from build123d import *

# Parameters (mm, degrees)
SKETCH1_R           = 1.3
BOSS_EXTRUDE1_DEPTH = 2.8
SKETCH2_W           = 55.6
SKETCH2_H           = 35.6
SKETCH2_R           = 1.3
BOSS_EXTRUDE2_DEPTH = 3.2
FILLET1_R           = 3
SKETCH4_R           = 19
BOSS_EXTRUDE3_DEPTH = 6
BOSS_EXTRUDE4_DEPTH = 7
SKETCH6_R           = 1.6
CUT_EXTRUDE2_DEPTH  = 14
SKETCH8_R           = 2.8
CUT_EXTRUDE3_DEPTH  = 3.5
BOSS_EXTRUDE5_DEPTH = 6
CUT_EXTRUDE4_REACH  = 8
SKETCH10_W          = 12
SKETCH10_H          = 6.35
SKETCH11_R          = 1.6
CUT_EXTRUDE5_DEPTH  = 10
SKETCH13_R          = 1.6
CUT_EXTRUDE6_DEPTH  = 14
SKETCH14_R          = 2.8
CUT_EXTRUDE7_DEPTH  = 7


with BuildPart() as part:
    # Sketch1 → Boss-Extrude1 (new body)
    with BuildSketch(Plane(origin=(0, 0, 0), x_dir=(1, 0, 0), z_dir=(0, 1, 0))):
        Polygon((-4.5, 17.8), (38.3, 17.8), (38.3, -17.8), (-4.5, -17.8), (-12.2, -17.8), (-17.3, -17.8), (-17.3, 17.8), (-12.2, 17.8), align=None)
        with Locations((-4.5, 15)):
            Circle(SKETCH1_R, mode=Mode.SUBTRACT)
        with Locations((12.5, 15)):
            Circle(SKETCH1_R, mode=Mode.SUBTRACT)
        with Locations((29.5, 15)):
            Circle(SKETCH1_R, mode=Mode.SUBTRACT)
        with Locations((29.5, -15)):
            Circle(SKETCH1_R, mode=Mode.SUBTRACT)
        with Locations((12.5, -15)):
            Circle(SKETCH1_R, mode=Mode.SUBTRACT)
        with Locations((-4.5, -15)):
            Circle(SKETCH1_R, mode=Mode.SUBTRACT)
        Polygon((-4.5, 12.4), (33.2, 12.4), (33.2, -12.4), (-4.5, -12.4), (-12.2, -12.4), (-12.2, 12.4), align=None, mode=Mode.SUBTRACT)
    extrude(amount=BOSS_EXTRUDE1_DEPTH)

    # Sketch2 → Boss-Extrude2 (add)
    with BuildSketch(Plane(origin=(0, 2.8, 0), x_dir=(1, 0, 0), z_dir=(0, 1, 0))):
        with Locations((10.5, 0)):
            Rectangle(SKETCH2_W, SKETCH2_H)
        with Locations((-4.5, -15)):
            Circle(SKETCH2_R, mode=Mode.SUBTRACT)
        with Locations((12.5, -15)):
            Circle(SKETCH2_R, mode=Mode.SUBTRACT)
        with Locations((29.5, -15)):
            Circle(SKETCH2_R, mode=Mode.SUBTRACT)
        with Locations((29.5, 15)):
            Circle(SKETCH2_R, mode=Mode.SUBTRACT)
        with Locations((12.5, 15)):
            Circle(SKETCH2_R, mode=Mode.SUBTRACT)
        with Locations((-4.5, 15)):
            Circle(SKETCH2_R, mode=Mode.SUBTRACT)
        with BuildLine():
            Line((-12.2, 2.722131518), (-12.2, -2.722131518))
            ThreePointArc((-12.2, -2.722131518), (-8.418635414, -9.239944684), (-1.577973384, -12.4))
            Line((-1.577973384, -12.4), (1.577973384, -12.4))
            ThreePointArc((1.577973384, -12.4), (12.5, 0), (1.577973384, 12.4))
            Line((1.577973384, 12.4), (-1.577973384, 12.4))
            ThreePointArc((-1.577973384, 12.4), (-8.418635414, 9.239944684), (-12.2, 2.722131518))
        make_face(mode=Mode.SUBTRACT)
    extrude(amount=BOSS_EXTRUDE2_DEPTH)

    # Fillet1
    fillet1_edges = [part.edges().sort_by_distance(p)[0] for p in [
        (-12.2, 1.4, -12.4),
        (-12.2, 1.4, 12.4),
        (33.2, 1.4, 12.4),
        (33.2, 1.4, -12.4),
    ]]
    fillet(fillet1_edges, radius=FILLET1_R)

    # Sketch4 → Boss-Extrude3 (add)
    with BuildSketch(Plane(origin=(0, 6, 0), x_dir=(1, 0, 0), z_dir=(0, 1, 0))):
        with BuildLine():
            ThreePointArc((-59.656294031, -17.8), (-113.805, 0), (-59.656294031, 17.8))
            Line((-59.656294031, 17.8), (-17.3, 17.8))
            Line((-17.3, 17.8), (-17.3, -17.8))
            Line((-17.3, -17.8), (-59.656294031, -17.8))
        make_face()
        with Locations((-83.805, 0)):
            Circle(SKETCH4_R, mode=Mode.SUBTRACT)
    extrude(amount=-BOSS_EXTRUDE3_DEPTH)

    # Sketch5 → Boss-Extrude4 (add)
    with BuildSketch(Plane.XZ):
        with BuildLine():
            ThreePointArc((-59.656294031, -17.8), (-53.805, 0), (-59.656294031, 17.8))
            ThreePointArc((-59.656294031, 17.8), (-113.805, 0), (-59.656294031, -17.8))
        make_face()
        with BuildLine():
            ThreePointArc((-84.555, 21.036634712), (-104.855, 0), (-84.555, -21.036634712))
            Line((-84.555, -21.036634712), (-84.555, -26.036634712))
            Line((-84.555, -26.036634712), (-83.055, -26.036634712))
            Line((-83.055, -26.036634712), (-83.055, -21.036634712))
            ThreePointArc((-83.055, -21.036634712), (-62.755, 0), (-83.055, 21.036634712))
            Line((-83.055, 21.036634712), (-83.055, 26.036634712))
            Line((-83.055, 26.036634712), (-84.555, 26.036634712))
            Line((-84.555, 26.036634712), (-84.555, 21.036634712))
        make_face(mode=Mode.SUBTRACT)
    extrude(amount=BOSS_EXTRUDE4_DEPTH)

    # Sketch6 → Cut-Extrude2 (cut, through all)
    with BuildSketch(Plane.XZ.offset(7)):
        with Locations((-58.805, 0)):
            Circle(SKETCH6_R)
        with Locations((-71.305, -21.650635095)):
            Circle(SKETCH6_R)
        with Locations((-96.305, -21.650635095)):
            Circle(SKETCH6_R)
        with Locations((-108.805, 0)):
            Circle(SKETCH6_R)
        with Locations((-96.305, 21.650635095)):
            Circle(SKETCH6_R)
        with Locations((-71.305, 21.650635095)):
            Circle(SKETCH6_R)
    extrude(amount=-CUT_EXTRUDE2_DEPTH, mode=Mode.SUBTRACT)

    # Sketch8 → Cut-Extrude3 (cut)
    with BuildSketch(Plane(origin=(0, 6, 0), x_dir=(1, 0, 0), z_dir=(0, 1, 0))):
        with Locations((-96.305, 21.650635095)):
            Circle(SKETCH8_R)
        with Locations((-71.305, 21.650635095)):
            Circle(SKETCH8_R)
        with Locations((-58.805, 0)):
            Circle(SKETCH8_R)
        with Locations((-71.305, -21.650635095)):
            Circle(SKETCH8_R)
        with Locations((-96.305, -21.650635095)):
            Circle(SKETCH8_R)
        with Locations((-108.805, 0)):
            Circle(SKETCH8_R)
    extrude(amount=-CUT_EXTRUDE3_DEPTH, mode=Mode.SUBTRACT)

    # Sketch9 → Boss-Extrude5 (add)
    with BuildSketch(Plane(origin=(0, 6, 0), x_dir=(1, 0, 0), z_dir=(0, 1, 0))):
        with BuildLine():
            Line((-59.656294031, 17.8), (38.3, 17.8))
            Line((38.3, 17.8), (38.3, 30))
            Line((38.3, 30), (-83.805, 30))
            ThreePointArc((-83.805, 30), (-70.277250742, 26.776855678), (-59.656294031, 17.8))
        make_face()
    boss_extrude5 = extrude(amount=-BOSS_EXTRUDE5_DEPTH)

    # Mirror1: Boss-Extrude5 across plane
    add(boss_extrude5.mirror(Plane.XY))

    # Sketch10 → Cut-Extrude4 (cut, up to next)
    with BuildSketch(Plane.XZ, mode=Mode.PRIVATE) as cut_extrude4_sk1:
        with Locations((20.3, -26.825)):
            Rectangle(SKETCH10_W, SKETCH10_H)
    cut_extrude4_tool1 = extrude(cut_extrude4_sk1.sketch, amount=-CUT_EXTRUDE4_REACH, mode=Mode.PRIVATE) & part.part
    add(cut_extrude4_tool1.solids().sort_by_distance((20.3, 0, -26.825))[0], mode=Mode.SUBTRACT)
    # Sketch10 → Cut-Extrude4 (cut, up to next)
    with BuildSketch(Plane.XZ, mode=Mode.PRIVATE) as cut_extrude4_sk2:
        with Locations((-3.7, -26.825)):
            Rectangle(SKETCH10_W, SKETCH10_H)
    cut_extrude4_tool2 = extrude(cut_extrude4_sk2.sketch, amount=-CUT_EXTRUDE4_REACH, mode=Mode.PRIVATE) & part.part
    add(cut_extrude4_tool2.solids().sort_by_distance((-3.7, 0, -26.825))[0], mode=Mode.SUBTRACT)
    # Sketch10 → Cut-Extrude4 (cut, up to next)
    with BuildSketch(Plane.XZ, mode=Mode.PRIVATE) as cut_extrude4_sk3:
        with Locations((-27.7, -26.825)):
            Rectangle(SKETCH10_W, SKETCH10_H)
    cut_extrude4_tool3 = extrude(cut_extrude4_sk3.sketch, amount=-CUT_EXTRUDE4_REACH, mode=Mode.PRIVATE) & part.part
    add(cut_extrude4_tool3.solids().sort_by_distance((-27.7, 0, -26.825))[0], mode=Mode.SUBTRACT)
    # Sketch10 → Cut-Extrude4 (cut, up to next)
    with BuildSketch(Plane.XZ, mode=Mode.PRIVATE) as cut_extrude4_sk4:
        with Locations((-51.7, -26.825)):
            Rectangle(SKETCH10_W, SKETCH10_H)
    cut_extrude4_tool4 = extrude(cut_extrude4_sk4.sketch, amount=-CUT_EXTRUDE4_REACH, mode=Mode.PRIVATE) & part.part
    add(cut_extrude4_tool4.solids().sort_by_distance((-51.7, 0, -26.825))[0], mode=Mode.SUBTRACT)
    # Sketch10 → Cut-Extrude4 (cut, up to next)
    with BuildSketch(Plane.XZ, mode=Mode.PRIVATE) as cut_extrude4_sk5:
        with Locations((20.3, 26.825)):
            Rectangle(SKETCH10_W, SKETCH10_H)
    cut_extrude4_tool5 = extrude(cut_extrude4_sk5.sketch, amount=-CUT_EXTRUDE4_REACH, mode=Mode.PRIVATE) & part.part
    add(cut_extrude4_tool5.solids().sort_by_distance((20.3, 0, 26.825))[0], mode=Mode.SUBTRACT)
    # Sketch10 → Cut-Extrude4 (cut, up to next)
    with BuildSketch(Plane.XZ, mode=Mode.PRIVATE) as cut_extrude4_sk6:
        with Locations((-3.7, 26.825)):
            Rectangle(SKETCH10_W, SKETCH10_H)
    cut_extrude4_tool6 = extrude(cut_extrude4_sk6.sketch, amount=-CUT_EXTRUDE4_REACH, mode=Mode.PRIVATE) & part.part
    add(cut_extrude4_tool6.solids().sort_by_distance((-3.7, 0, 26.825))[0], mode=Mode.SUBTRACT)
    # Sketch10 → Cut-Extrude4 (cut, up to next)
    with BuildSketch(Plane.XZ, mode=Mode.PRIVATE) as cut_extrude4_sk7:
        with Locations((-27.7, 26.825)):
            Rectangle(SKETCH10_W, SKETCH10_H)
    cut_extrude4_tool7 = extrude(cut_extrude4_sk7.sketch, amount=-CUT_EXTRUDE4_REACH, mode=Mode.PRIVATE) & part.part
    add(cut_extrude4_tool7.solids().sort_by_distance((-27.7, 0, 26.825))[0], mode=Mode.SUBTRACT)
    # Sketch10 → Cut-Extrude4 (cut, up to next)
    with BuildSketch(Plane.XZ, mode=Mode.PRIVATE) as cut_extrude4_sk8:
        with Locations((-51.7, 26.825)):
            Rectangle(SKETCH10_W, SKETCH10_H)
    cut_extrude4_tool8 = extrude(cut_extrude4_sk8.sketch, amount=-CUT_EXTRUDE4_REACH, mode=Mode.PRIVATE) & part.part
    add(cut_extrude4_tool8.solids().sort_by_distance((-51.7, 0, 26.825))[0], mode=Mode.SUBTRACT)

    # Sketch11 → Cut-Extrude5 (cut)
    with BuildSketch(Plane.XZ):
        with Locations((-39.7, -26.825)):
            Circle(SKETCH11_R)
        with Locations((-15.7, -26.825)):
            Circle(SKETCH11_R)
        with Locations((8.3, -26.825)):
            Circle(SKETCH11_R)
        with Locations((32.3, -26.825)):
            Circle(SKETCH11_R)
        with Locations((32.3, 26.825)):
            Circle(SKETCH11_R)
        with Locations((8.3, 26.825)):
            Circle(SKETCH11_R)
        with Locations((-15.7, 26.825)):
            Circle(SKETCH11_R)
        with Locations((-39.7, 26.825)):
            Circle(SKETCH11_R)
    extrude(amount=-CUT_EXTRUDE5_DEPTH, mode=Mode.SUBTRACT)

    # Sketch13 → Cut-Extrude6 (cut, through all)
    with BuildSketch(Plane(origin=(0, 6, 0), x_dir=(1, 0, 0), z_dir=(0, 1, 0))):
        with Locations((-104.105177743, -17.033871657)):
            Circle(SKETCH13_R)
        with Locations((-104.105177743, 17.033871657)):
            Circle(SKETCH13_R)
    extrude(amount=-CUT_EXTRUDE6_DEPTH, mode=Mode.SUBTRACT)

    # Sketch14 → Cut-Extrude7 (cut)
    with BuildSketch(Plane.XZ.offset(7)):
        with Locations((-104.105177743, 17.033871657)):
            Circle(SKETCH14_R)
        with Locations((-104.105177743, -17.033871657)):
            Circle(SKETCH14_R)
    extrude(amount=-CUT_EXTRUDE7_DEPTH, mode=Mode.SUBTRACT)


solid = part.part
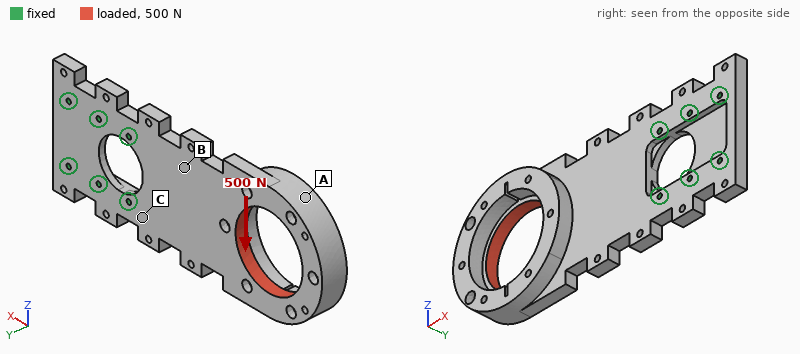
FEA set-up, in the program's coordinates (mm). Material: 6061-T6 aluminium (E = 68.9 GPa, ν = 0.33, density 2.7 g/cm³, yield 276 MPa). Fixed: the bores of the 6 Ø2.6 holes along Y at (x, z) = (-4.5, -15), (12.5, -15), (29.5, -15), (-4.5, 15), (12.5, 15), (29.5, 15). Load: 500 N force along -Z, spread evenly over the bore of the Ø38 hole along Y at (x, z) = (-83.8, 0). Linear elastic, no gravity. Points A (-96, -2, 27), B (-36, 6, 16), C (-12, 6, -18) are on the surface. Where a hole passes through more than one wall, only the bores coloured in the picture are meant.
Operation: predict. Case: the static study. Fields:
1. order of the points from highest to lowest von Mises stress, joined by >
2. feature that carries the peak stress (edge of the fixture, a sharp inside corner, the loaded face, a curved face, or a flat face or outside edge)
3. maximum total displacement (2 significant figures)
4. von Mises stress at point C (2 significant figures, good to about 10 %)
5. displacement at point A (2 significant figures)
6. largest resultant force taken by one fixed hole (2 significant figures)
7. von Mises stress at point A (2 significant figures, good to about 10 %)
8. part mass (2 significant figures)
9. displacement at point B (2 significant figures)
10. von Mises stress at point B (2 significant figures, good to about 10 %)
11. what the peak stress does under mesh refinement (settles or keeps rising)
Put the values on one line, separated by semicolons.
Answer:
C > B > A; edge of the fixture; 64 µm; 12 MPa; 54 µm; 930 N; 2.9 MPa; 120 g; 12 µm; 7.4 MPa; keeps rising
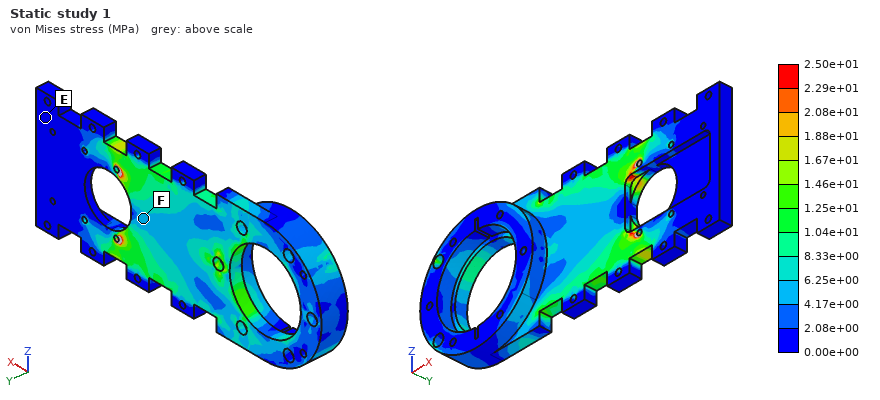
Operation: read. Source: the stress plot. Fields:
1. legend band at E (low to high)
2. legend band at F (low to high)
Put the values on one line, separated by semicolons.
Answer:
0.00e+00 to 2.08e+00 MPa; 4.17e+00 to 6.25e+00 MPa
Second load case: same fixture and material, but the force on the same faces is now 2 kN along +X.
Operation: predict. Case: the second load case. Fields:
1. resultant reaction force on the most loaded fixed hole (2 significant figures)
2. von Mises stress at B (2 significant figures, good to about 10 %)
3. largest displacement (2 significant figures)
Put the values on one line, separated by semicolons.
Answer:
870 N; 7.8 MPa; 25 µm
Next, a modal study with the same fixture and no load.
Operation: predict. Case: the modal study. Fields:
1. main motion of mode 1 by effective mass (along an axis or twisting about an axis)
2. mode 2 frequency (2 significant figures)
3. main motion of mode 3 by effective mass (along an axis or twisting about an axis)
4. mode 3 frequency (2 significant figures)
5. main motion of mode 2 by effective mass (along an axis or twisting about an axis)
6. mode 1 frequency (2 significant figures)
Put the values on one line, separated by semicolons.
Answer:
along Y; 1400 Hz; along Z; 2200 Hz; twisting about X; 340 Hz
